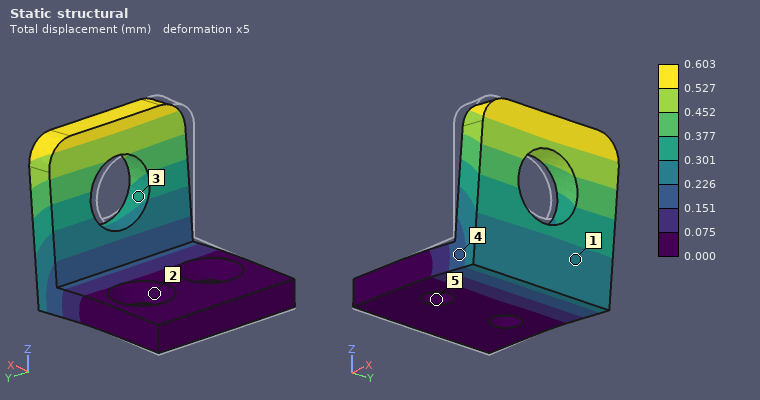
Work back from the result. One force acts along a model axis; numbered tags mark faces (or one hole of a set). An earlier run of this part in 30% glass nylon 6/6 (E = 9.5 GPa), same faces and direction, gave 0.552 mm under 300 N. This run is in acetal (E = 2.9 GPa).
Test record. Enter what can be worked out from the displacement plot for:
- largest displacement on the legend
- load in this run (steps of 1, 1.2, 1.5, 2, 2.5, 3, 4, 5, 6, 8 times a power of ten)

0.603 mm
100 N
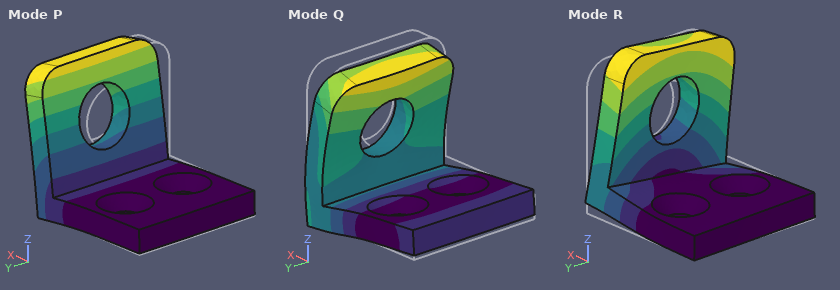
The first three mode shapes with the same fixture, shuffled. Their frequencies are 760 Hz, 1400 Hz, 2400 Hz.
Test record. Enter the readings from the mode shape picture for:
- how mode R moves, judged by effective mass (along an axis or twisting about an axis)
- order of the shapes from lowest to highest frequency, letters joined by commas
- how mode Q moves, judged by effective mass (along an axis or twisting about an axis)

along Y
P, R, Q
along Z
